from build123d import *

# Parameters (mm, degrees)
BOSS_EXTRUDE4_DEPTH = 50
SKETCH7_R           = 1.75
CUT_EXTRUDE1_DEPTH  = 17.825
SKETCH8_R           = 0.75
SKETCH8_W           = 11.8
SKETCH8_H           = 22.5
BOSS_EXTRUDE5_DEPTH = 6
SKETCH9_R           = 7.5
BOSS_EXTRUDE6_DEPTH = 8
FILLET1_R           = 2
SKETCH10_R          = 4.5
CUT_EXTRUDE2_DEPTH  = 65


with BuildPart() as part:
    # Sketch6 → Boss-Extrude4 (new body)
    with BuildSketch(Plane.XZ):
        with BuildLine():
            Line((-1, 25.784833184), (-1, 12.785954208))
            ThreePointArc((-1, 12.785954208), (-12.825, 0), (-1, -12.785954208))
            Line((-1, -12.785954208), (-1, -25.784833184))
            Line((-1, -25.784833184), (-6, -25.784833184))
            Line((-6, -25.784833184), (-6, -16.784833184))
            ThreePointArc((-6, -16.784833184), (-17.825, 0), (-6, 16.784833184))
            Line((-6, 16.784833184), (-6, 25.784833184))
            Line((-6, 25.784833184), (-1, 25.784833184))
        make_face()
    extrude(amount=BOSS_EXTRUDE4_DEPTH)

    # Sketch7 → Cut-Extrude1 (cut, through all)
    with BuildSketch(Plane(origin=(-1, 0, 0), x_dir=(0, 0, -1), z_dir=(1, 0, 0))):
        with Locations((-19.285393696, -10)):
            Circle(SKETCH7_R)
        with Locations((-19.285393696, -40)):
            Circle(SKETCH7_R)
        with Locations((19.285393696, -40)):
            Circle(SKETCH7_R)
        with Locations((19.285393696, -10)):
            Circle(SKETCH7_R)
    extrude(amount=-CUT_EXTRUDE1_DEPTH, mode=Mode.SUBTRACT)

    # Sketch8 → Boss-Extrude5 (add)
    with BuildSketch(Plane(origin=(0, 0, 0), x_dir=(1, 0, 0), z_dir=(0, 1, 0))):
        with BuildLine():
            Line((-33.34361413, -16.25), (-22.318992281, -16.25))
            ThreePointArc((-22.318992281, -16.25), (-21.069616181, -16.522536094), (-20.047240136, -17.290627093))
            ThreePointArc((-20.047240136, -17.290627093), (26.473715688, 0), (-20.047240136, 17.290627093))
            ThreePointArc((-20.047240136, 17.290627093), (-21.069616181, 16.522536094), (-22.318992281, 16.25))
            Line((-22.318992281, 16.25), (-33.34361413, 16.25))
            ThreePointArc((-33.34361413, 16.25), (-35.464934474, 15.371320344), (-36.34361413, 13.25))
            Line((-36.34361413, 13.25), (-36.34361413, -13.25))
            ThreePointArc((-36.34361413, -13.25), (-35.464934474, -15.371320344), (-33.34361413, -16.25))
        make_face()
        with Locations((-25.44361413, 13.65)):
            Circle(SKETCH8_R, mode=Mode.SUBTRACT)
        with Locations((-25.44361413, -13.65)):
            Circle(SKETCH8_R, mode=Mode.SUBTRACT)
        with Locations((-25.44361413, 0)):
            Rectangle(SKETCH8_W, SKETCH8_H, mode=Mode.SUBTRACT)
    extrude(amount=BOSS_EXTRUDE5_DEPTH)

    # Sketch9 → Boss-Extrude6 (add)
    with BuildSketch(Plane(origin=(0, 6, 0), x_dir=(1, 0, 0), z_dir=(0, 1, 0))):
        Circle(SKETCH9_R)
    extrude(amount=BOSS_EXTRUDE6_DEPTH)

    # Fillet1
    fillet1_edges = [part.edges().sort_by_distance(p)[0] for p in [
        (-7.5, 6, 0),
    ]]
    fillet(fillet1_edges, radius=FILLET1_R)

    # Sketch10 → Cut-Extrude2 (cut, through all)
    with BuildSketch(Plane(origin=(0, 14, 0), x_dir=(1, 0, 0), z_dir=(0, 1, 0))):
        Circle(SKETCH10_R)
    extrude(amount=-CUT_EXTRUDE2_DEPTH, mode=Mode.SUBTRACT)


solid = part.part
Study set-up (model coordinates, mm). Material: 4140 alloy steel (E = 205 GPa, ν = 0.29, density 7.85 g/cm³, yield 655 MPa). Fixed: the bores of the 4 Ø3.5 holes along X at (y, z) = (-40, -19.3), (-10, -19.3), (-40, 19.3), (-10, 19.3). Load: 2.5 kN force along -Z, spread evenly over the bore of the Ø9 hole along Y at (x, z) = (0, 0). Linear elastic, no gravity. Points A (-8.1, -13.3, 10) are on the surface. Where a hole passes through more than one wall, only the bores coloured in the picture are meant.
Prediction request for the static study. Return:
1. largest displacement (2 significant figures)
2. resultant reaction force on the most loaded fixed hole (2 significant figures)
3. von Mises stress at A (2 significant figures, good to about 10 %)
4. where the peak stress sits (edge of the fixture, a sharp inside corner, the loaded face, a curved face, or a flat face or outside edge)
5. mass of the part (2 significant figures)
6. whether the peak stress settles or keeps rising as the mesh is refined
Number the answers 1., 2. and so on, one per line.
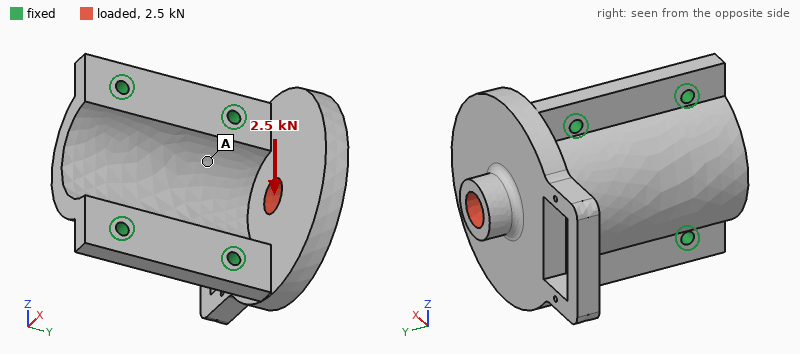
1. 10 µm
2. 1.5 kN
3. 9.9 MPa
4. edge of the fixture
5. 240 g
6. keeps rising
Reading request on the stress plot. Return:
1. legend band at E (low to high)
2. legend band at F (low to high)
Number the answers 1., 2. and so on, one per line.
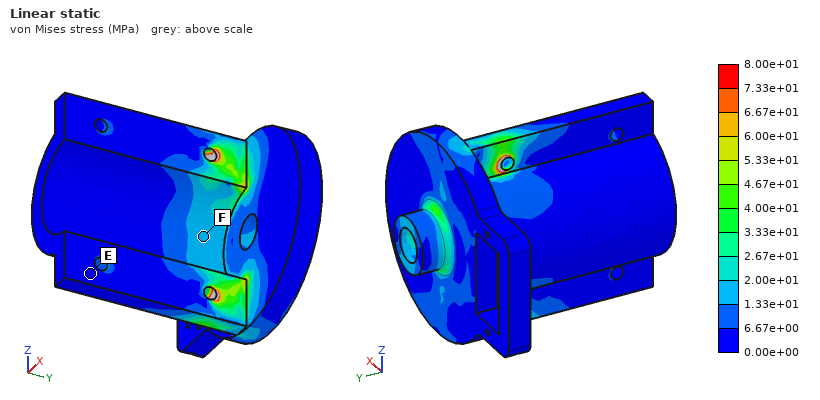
1. 0.00e+00 to 6.67e+00 MPa
2. 1.33e+01 to 2.00e+01 MPa
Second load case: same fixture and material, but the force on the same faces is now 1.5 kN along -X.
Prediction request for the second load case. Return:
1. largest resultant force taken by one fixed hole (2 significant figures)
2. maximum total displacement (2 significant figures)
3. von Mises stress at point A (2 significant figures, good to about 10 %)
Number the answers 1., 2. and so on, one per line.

1. 1.4 kN
2. 23 µm
3. 9.6 MPa
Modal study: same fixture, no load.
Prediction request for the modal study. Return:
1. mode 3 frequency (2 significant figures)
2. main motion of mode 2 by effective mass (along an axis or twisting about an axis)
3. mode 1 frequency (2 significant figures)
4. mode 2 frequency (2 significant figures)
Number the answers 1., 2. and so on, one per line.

1. 7000 Hz
2. along Y
3. 4200 Hz
4. 6300 Hz
